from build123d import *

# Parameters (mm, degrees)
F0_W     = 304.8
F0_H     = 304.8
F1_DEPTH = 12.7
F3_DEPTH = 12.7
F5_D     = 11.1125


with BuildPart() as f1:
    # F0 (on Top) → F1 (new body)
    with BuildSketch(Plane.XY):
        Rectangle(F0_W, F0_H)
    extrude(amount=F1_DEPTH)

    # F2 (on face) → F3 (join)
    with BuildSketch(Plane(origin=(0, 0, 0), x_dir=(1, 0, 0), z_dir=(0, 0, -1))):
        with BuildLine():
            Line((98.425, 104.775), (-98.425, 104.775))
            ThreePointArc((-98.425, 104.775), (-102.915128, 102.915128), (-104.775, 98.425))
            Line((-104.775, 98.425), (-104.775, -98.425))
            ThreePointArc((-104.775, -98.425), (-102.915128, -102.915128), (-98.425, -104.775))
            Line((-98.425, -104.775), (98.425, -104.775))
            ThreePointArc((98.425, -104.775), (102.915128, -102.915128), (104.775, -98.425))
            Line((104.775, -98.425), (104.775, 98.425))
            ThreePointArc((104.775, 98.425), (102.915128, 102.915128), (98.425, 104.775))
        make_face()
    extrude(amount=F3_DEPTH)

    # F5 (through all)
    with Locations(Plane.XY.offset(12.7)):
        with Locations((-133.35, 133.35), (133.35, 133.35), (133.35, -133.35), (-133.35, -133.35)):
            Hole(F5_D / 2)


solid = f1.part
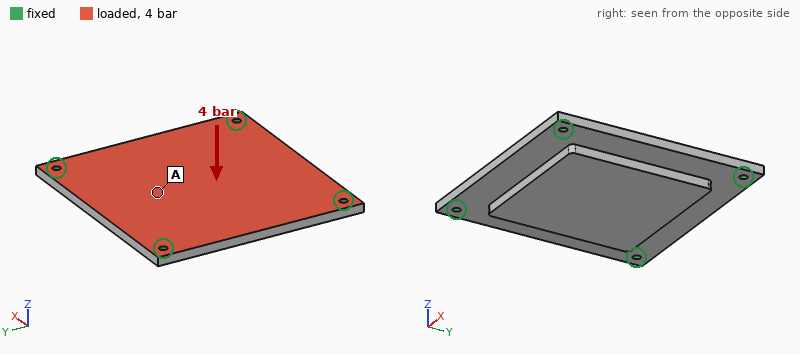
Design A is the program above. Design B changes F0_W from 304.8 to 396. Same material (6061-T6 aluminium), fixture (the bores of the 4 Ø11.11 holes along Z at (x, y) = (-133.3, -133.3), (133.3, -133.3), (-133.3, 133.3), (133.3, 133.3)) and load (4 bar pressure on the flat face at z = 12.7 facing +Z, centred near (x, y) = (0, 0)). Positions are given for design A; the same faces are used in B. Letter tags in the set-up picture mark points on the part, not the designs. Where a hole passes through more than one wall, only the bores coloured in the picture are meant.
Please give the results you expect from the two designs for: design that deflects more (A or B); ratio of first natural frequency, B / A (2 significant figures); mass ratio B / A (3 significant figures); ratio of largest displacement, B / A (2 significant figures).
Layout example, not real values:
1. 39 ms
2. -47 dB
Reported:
1. B
2. 1.0
3. 1.20
4. 1.2
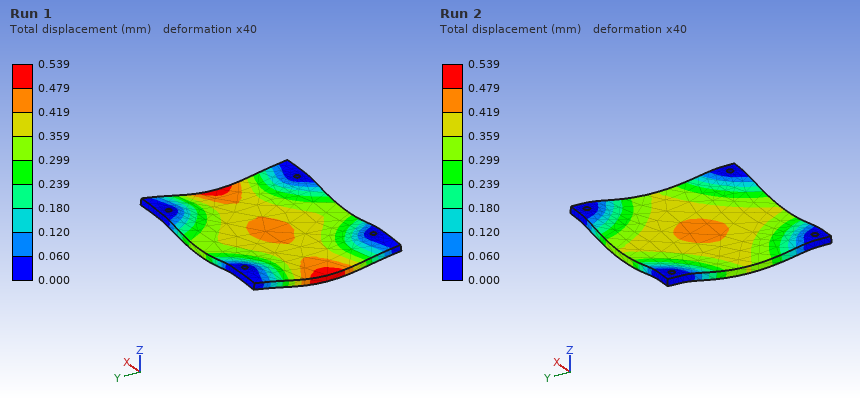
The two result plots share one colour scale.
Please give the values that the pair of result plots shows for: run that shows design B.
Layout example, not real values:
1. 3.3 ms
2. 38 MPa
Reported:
1. Run 1
